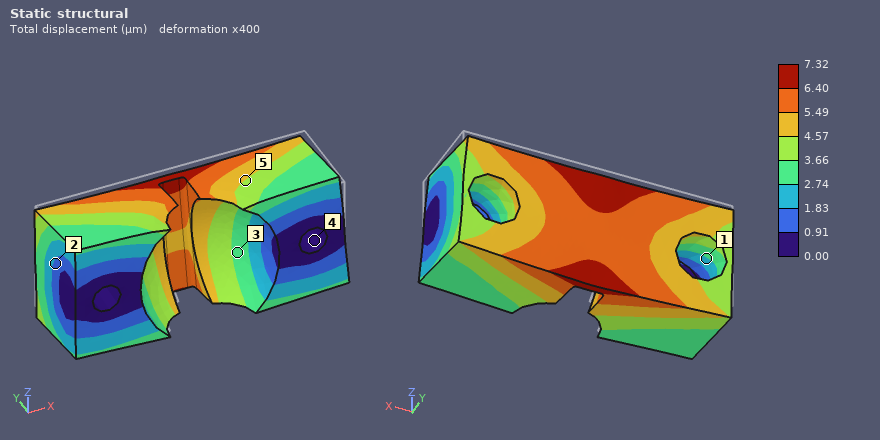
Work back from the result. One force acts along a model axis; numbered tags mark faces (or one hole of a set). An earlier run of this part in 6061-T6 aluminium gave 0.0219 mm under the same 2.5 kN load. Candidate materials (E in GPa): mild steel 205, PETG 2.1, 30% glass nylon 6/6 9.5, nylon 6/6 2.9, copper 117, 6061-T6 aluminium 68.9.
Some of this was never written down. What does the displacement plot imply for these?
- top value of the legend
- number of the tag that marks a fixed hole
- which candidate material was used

7.32 µm
4
mild steel
